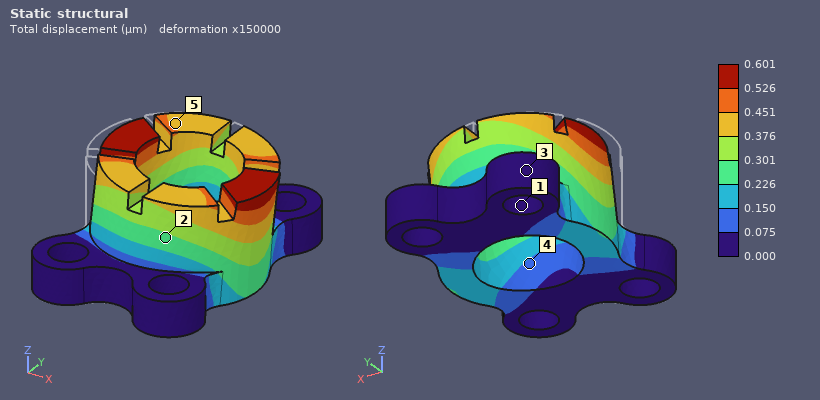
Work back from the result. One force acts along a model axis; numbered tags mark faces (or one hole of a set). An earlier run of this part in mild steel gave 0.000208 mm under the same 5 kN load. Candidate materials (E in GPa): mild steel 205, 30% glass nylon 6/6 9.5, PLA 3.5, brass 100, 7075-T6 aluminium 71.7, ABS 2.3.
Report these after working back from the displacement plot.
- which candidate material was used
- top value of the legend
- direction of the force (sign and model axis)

7075-T6 aluminium
0.601 µm
+X
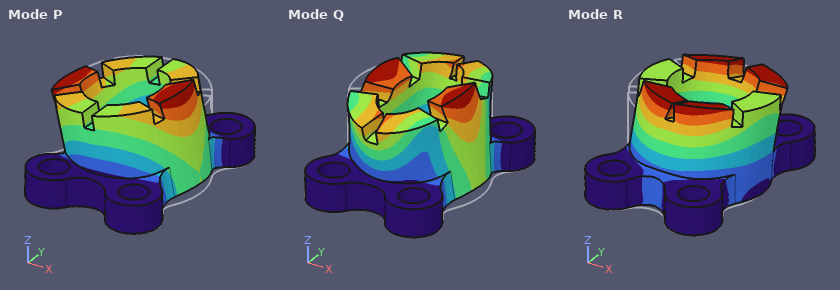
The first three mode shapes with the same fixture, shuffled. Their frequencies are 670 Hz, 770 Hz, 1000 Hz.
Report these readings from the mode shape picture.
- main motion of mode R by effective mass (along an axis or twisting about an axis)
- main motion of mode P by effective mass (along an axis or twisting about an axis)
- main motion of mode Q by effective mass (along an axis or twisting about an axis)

along Y
along X
along Z
